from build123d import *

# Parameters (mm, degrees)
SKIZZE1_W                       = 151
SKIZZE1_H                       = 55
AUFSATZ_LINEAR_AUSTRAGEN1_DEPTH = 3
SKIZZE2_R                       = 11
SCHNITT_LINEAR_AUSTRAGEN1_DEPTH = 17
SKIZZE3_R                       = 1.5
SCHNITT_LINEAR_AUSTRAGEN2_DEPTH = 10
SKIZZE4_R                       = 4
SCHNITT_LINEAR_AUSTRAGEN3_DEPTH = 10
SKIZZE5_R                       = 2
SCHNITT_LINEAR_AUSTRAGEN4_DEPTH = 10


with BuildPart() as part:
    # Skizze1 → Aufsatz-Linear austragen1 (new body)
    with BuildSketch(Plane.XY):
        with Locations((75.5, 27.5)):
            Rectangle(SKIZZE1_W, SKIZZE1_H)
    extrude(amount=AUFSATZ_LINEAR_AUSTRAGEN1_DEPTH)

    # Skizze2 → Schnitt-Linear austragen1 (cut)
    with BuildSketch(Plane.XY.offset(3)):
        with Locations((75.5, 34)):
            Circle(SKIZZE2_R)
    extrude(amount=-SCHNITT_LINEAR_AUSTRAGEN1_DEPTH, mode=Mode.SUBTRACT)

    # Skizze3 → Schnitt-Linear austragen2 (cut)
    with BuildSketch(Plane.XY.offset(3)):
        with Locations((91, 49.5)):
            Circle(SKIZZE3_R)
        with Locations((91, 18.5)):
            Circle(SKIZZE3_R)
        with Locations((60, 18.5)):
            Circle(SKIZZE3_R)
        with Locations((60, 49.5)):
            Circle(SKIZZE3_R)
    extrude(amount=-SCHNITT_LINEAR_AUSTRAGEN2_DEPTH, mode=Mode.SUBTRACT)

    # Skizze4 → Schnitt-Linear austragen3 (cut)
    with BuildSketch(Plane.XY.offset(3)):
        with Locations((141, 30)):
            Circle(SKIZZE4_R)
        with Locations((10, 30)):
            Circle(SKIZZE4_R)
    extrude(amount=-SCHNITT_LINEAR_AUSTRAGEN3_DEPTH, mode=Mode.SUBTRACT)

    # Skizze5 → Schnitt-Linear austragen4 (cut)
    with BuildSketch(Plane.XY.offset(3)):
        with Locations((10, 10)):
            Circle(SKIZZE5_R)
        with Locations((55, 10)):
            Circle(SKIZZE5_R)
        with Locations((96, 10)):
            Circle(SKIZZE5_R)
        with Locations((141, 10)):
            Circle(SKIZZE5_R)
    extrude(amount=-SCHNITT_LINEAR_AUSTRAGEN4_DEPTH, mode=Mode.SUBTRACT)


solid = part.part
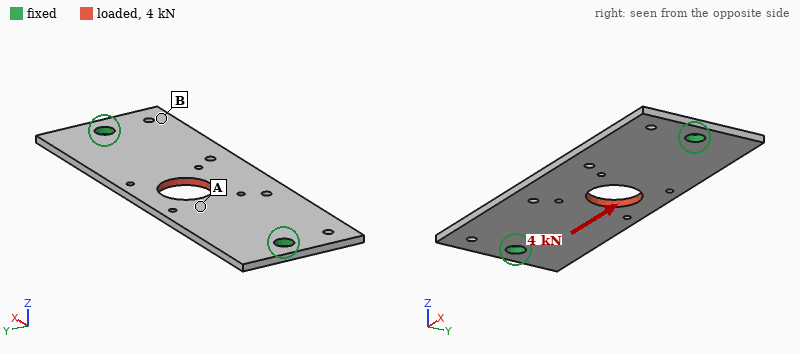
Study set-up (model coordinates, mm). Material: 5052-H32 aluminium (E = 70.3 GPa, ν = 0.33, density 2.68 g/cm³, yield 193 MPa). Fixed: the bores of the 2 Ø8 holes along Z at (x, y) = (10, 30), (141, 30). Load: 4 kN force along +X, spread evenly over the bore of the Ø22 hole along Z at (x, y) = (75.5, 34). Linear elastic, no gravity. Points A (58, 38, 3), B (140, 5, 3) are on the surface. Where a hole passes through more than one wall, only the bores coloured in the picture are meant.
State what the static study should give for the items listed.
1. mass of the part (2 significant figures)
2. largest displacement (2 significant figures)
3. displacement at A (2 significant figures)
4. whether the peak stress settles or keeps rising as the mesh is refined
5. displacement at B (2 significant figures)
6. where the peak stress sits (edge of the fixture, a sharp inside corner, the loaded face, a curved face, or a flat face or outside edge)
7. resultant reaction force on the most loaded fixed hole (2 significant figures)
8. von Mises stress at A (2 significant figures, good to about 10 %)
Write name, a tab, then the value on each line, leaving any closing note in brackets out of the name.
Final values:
mass of the part	62 g
largest displacement	19 µm
displacement at A	15 µm
whether the peak stress settles or keeps rising as the mesh is refined	keeps rising
displacement at B	8.1 µm
where the peak stress sits	edge of the fixture
resultant reaction force on the most loaded fixed hole	2.0 kN
von Mises stress at A	20 MPa
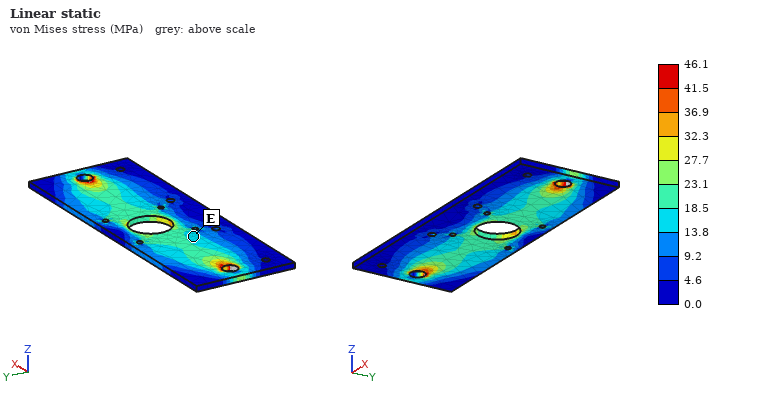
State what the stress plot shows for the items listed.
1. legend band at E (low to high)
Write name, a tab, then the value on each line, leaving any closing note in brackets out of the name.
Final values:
legend band at E	13.8 to 18.5 MPa
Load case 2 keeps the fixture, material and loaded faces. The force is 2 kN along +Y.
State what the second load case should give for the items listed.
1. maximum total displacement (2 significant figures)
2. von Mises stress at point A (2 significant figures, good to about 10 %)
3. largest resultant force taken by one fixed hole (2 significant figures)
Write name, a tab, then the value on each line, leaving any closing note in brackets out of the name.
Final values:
maximum total displacement	45 µm
von Mises stress at point A	17 MPa
largest resultant force taken by one fixed hole	1.0 kN
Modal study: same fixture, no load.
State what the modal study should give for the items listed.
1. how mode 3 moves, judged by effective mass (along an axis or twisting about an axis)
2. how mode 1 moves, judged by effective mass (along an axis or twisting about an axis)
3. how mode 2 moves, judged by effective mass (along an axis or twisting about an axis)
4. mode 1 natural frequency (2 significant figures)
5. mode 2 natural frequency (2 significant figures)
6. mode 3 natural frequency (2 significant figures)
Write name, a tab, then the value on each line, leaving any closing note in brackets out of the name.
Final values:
how mode 3 moves, judged by effective mass	twisting about Y
how mode 1 moves, judged by effective mass	along Z
how mode 2 moves, judged by effective mass	twisting about X
mode 1 natural frequency	900 Hz
mode 2 natural frequency	1300 Hz
mode 3 natural frequency	2300 Hz
